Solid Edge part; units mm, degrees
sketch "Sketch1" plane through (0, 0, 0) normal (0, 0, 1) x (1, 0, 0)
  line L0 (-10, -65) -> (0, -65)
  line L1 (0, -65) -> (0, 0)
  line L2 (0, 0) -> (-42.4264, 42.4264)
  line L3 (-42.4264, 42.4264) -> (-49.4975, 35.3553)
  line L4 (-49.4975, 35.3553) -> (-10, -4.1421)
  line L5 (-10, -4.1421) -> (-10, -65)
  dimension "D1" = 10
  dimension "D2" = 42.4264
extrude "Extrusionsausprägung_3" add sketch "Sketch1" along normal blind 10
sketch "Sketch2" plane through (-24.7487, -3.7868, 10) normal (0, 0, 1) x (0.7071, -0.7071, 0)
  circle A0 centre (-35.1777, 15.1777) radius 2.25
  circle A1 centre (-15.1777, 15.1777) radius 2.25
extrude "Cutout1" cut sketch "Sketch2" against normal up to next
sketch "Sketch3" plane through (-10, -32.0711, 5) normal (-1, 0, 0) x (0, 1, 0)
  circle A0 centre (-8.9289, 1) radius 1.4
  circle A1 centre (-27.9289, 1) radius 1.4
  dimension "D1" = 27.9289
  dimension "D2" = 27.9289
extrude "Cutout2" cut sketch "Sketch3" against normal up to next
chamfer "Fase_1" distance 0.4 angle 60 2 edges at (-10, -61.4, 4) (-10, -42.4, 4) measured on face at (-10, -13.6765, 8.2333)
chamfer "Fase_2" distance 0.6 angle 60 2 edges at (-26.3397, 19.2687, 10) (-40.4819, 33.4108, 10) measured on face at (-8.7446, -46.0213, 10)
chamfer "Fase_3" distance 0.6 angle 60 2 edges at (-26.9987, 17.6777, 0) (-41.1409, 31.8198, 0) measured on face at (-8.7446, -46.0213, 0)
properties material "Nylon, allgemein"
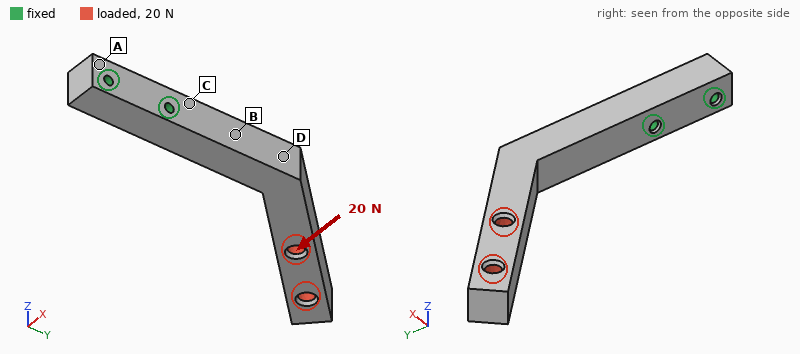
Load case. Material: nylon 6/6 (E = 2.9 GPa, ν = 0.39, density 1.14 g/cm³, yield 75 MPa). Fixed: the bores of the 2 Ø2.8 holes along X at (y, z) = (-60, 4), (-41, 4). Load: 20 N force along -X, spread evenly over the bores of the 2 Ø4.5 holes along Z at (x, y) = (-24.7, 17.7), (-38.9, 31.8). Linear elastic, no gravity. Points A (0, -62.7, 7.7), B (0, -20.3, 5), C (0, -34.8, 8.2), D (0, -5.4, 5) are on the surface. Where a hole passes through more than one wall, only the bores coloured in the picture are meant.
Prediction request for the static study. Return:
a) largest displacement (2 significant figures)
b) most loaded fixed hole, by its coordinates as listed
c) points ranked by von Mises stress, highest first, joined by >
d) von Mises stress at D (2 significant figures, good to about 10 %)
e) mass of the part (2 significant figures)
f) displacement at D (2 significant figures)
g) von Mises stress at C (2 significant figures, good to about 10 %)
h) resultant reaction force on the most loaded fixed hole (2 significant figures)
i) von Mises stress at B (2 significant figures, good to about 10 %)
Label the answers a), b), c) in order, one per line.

a) 1.4 mm
b) (-41, 4)
c) C > B > D > A
d) 3.2 MPa
e) 13 g
f) 0.31 mm
g) 6.7 MPa
h) 33 N
i) 5.4 MPa
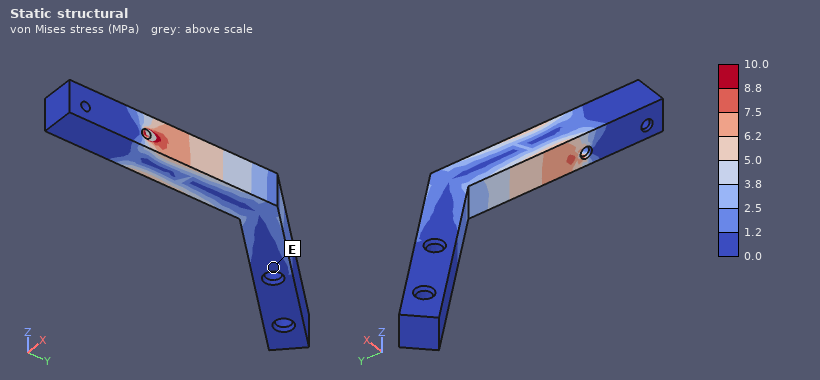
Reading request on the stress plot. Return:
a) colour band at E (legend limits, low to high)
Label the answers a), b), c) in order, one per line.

a) 0.0 to 1.2 MPa
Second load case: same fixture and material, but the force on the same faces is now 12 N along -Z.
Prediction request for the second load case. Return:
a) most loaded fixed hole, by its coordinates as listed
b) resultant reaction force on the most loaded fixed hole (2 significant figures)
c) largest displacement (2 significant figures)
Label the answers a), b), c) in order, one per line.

a) (-41, 4)
b) 43 N
c) 1.2 mm
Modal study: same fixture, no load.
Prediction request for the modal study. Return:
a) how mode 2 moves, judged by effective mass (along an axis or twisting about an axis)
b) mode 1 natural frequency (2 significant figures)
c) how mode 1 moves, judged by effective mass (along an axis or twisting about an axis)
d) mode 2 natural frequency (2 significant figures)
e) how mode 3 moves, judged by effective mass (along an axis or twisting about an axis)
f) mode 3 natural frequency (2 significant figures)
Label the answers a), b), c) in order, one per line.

a) along X
b) 270 Hz
c) along Z
d) 300 Hz
e) along Z
f) 1200 Hz
